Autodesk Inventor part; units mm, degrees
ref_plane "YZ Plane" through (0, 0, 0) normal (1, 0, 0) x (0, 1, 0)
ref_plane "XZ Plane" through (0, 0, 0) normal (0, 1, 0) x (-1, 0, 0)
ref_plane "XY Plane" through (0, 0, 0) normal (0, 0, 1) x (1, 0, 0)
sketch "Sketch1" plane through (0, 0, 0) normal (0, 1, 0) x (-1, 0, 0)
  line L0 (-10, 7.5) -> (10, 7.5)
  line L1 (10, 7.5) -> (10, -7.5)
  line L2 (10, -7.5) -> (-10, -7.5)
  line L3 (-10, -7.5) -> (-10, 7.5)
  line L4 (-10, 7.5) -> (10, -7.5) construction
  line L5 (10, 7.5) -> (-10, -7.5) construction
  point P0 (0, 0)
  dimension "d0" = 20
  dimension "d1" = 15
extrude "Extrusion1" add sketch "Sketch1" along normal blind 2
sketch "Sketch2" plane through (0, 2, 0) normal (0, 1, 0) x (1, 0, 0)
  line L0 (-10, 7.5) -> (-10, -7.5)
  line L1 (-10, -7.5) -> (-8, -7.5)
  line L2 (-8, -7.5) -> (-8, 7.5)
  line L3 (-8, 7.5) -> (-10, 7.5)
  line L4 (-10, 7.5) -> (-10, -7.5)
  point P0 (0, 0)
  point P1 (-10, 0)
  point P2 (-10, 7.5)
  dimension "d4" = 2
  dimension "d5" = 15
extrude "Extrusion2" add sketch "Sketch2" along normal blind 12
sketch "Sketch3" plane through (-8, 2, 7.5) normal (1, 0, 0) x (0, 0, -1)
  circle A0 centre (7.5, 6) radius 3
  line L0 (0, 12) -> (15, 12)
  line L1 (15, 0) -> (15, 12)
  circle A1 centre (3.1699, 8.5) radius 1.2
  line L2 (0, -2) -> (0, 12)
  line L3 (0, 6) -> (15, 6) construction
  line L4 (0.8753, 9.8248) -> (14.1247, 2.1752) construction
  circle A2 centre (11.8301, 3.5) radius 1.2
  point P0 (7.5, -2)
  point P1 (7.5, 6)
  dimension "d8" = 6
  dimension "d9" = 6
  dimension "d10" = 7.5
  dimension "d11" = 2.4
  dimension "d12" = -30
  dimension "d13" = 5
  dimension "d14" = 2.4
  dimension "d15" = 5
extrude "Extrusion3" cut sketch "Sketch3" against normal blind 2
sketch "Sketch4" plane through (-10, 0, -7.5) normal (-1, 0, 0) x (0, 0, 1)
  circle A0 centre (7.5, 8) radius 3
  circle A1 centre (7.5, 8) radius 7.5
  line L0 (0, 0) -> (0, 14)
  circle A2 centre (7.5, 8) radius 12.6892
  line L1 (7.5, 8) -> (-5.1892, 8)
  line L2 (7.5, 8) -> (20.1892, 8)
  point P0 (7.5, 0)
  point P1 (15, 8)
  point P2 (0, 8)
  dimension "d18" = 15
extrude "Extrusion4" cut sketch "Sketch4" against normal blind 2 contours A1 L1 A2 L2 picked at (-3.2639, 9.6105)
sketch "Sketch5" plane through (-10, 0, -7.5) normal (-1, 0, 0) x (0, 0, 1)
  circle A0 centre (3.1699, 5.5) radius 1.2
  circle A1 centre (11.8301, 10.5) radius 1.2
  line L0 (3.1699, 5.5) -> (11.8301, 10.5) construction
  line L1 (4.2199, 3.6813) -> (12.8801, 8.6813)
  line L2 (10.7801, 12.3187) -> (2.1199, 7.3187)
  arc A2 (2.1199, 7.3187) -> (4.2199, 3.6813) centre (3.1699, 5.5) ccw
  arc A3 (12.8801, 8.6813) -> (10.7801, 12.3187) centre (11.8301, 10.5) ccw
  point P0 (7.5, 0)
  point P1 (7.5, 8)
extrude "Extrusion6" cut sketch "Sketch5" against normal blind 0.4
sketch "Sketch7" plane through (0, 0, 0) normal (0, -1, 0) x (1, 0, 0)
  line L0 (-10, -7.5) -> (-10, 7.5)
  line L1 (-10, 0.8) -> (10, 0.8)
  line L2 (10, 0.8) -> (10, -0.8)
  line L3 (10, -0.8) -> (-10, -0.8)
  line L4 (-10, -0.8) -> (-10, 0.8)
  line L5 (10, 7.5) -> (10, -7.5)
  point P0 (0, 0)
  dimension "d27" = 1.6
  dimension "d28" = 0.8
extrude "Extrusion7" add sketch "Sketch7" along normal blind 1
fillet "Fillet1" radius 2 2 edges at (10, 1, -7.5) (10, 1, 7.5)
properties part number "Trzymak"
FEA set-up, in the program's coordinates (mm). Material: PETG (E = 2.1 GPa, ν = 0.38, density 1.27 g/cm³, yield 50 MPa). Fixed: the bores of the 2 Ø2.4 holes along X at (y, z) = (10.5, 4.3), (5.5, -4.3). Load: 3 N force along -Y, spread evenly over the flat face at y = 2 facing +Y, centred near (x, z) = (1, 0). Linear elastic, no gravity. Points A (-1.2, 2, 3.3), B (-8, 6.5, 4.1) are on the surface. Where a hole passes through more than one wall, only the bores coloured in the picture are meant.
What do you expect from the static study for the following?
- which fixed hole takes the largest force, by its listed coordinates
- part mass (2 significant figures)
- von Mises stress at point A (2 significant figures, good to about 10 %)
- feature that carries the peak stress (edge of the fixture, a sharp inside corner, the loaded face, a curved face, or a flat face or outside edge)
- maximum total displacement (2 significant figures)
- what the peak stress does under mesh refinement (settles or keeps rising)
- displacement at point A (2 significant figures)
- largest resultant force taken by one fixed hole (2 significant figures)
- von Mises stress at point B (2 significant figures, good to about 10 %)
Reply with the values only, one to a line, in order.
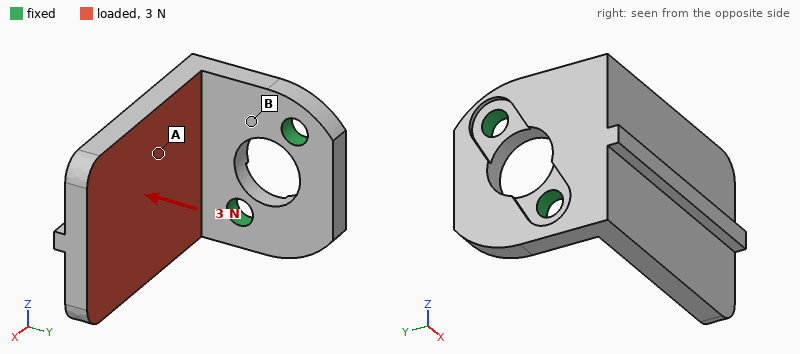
(5.5, -4.3)
1.1 g
0.81 MPa
edge of the fixture
0.28 mm
keeps rising
0.10 mm
2.1 N
2.8 MPa
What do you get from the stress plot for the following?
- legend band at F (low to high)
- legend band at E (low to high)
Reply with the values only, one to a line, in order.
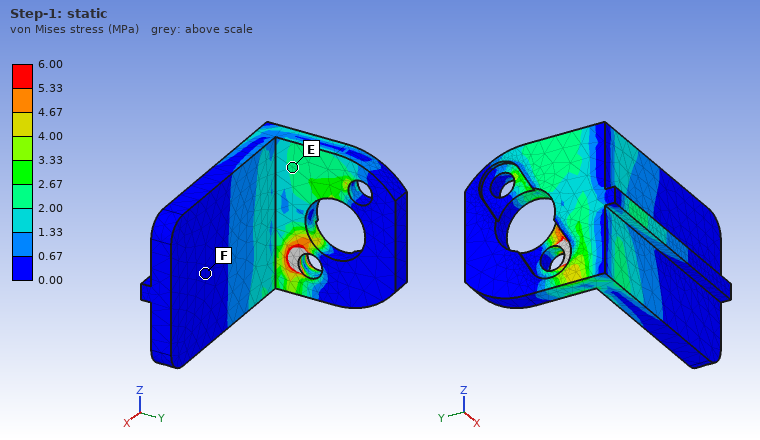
0.00 to 0.67 MPa
2.00 to 2.67 MPa
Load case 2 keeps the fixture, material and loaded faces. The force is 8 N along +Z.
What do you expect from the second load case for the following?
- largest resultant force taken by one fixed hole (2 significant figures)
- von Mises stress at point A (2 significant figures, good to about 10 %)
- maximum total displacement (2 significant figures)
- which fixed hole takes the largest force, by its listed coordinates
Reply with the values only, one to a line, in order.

8.7 N
1.2 MPa
0.29 mm
(5.5, -4.3)
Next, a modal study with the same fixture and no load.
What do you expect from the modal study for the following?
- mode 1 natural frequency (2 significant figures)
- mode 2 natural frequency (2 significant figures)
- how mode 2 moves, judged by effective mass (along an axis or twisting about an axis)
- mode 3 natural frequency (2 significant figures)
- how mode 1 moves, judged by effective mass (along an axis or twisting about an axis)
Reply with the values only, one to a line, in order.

730 Hz
1400 Hz
along Z
3100 Hz
along Y
